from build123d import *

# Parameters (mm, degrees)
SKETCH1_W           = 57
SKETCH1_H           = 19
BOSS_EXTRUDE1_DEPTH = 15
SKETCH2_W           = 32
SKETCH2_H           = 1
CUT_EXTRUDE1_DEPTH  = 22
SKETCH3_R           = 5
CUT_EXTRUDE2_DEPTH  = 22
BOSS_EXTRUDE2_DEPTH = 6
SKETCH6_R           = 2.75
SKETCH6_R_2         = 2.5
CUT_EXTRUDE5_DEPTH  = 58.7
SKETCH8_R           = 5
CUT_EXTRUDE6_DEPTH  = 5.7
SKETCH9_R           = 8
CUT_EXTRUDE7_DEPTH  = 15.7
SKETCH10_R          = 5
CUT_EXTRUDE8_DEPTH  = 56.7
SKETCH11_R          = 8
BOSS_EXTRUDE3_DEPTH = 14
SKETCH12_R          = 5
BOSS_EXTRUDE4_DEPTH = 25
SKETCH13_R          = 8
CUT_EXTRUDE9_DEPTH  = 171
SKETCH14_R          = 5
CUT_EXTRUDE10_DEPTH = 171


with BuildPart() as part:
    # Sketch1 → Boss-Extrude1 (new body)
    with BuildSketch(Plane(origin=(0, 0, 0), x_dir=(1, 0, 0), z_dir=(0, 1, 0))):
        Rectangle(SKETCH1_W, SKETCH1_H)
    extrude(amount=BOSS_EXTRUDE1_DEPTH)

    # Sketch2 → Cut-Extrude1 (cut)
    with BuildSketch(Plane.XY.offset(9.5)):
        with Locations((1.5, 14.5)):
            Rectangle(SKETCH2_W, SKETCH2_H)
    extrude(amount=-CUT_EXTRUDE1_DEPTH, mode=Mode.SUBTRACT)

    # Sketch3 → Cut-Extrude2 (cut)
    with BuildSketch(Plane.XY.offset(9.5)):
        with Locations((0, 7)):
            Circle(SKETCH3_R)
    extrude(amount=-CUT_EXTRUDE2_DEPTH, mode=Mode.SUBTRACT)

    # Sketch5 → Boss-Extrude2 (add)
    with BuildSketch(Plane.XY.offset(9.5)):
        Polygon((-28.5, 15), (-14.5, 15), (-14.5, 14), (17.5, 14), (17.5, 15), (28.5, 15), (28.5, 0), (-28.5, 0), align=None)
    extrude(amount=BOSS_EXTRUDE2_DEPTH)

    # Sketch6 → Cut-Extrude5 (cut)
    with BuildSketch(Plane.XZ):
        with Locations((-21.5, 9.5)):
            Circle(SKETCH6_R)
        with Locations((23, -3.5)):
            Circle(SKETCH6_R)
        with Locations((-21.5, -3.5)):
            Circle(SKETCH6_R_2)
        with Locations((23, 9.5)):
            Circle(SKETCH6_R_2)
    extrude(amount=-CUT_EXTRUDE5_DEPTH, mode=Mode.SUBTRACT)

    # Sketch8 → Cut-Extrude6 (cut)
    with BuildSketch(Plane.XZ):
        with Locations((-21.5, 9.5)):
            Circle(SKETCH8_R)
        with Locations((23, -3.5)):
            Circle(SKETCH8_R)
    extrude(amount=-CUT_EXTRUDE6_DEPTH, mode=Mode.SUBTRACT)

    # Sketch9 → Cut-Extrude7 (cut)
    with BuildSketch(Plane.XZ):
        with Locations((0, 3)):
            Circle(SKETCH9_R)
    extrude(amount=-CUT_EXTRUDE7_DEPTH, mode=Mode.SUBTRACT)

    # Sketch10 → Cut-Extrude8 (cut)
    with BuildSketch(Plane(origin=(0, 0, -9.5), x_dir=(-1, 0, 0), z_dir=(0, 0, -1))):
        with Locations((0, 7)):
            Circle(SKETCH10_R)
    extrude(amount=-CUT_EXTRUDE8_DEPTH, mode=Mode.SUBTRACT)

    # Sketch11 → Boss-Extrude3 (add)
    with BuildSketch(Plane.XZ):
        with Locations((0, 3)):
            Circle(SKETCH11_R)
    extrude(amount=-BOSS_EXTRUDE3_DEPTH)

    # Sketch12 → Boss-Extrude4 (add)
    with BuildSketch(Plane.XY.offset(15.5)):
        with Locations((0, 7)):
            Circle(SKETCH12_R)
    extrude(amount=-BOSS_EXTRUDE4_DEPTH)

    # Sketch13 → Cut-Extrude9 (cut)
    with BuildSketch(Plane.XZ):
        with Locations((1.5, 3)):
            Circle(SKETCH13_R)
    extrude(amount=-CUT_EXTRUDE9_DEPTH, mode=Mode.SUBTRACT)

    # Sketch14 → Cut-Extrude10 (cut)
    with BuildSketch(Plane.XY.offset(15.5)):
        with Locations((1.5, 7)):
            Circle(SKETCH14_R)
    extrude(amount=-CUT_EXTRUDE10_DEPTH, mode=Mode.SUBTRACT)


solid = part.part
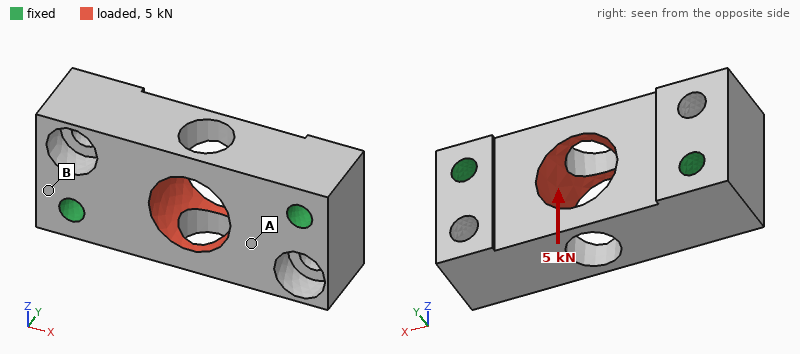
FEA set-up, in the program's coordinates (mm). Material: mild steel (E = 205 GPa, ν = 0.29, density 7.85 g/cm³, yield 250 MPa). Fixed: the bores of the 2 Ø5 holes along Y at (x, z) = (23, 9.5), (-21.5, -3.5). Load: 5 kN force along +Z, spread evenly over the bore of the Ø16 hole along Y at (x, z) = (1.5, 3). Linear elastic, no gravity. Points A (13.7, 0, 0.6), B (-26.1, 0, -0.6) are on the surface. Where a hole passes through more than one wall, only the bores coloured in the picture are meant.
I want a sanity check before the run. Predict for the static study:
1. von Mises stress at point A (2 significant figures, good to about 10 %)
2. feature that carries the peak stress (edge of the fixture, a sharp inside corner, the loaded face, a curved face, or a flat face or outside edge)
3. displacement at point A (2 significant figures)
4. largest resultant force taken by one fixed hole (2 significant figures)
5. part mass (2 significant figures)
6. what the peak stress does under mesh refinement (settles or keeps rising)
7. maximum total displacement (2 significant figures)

16 MPa
a sharp inside corner
3.4 µm
2.6 kN
120 g
keeps rising
6.6 µm
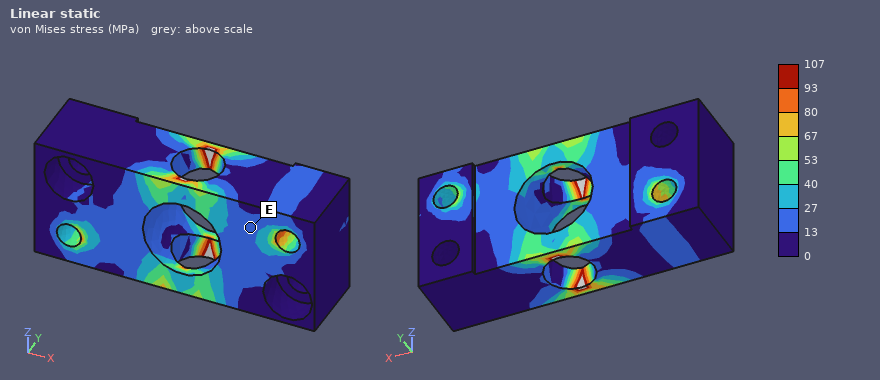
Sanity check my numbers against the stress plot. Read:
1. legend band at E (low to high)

13 to 27 MPa
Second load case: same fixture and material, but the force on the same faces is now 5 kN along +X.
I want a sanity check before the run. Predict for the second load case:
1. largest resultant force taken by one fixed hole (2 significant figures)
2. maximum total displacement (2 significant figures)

2.5 kN
2.6 µm
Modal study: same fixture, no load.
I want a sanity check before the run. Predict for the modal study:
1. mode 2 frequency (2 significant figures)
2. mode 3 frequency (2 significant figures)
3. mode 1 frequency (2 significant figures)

20 kHz
21 kHz
20 kHz
